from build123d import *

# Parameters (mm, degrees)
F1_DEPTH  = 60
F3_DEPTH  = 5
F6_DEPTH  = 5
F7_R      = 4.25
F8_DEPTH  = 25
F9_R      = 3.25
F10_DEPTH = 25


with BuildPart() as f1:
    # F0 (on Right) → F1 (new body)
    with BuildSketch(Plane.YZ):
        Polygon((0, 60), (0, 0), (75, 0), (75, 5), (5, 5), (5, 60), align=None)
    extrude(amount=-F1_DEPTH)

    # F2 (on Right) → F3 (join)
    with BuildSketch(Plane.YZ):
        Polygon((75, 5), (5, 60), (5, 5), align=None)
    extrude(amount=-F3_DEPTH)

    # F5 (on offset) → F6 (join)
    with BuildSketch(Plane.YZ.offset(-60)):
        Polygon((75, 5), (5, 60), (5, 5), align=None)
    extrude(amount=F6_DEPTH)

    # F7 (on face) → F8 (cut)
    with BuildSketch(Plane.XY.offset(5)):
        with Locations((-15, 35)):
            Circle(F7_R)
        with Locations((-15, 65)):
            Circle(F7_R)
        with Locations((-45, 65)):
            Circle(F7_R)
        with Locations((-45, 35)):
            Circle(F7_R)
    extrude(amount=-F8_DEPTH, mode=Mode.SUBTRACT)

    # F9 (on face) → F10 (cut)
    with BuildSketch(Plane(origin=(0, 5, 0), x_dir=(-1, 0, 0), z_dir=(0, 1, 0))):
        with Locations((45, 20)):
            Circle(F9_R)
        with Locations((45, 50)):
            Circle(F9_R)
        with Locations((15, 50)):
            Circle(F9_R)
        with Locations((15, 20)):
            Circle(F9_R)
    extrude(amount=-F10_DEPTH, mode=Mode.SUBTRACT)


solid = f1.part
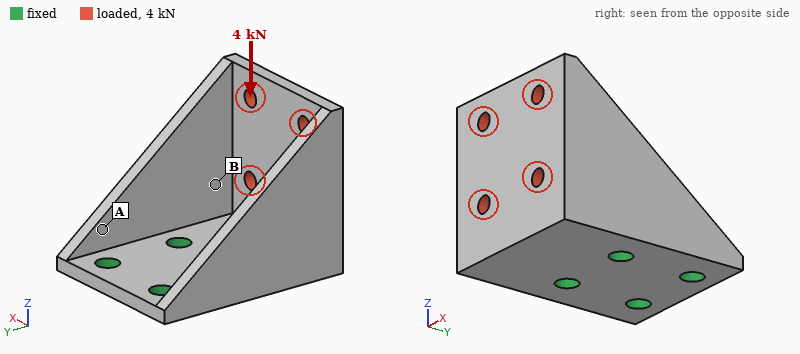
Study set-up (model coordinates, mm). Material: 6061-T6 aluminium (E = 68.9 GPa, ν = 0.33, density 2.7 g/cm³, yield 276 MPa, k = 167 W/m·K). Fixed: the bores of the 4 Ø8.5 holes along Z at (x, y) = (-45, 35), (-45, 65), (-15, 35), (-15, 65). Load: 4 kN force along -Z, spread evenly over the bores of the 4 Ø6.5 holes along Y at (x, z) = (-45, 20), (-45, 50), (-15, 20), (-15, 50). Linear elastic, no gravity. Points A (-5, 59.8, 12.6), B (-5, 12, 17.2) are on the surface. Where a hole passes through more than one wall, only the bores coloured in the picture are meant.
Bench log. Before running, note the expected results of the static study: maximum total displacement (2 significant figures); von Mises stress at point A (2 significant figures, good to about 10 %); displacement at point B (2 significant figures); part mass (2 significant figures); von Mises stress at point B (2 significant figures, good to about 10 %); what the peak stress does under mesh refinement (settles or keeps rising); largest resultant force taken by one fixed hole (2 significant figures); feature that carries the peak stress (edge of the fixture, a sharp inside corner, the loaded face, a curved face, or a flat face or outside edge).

0.23 mm
62 MPa
0.12 mm
150 g
27 MPa
keeps rising
3.6 kN
edge of the fixture
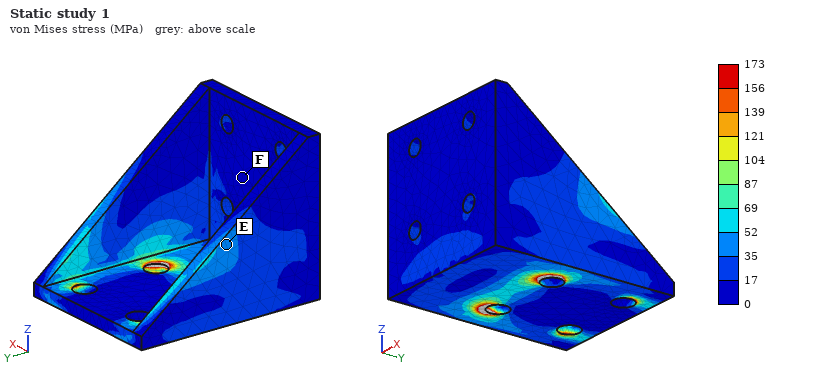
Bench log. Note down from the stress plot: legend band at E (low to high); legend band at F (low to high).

35 to 52 MPa
0 to 17 MPa
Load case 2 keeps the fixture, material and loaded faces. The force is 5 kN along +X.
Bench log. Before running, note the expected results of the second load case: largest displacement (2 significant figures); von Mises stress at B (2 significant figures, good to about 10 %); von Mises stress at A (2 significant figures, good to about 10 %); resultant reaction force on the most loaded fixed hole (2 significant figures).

0.67 mm
39 MPa
110 MPa
6.9 kN
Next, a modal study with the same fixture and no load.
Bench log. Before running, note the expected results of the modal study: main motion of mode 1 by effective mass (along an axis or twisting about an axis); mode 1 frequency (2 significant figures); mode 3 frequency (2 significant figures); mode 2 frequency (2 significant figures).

along X
1900 Hz
4400 Hz
2500 Hz
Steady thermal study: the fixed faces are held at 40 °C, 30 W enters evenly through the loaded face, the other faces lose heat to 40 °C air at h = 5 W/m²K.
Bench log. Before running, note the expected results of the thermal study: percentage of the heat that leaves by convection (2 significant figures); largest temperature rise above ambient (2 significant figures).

3.4 %
21 K
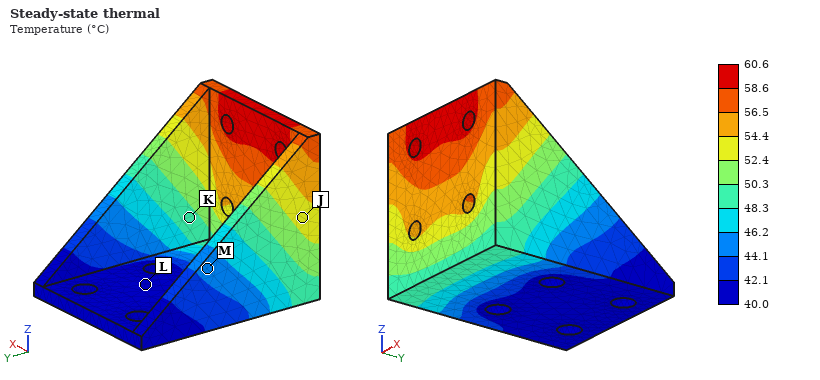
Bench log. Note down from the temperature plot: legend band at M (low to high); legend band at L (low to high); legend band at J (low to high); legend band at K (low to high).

44.1 to 46.2 °C
40.0 to 42.1 °C
52.4 to 54.4 °C
48.3 to 50.3 °C
